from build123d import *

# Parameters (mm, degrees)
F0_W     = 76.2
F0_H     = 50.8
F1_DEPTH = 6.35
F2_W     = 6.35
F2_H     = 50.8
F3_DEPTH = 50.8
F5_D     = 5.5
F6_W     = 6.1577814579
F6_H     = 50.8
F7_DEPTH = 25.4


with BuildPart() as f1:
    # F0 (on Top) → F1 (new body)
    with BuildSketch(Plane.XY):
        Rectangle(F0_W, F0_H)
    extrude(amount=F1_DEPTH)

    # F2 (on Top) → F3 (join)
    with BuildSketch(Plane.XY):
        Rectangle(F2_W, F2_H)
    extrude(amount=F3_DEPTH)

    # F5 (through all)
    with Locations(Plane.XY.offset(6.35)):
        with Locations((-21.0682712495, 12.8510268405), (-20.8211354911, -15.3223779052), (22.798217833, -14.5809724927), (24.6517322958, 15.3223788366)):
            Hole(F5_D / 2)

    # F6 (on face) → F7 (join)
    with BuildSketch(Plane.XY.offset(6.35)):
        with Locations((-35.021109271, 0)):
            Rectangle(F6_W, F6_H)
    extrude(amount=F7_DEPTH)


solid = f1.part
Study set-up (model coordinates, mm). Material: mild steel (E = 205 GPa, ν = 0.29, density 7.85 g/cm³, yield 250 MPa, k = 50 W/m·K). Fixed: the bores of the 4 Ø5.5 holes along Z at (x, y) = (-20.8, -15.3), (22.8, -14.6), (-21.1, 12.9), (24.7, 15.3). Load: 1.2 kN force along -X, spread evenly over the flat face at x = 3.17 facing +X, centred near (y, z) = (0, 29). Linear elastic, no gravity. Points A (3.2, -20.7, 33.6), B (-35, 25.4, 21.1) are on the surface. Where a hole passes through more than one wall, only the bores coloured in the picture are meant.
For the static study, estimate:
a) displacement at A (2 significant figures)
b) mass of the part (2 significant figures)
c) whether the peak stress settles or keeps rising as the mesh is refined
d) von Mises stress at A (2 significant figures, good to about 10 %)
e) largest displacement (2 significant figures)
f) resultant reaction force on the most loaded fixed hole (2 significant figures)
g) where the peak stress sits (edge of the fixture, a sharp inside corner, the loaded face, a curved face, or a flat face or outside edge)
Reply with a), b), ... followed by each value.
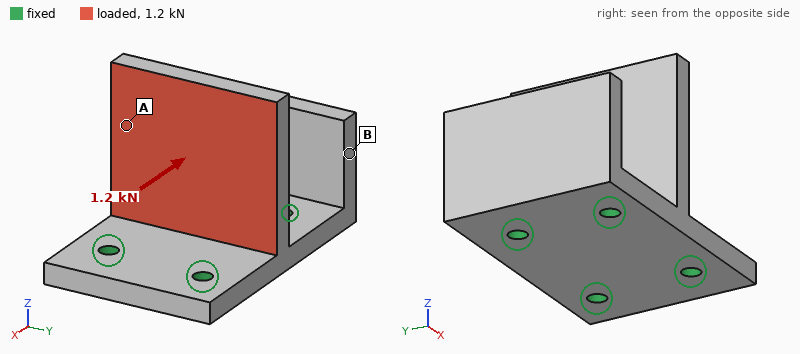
a) 43 µm
b) 360 g
c) keeps rising
d) 12 MPa
e) 82 µm
f) 600 N
g) edge of the fixture
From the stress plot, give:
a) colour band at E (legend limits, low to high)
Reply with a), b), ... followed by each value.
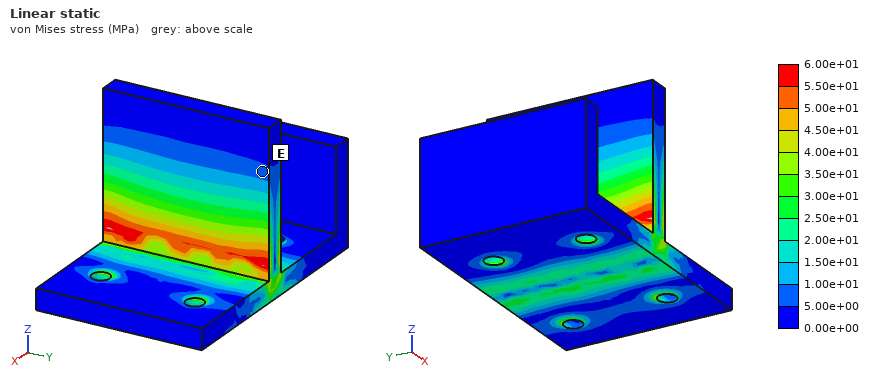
a) 5.00e+00 to 1.00e+01 MPa
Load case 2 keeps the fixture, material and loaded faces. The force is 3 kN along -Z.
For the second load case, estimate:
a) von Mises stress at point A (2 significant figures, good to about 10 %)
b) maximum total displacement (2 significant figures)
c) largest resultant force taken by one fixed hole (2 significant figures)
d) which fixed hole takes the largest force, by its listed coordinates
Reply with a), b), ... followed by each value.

a) 15 MPa
b) 39 µm
c) 900 N
d) (22.8, -14.6)
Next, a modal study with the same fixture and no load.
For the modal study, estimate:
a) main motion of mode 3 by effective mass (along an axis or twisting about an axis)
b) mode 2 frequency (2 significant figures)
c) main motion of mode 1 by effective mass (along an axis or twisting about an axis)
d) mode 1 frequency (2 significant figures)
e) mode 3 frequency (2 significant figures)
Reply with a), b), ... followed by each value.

a) along Y
b) 3700 Hz
c) along X
d) 2300 Hz
e) 4600 Hz
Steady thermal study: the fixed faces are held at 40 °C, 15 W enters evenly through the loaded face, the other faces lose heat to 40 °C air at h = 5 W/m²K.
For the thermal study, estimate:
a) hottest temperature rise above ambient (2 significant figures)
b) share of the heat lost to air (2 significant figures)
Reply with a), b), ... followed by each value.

a) 31 K
b) 3.7 %
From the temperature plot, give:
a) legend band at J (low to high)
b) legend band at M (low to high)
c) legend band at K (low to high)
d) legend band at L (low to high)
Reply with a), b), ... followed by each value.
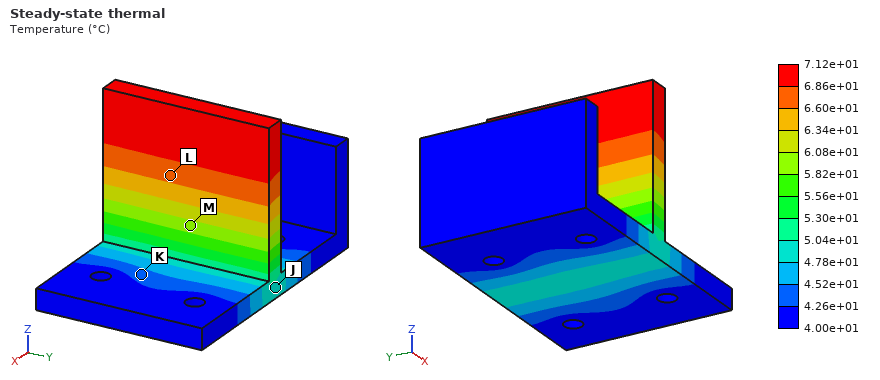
a) 4.78e+01 to 5.04e+01 °C
b) 5.82e+01 to 6.08e+01 °C
c) 4.26e+01 to 4.52e+01 °C
d) 6.60e+01 to 6.86e+01 °C
